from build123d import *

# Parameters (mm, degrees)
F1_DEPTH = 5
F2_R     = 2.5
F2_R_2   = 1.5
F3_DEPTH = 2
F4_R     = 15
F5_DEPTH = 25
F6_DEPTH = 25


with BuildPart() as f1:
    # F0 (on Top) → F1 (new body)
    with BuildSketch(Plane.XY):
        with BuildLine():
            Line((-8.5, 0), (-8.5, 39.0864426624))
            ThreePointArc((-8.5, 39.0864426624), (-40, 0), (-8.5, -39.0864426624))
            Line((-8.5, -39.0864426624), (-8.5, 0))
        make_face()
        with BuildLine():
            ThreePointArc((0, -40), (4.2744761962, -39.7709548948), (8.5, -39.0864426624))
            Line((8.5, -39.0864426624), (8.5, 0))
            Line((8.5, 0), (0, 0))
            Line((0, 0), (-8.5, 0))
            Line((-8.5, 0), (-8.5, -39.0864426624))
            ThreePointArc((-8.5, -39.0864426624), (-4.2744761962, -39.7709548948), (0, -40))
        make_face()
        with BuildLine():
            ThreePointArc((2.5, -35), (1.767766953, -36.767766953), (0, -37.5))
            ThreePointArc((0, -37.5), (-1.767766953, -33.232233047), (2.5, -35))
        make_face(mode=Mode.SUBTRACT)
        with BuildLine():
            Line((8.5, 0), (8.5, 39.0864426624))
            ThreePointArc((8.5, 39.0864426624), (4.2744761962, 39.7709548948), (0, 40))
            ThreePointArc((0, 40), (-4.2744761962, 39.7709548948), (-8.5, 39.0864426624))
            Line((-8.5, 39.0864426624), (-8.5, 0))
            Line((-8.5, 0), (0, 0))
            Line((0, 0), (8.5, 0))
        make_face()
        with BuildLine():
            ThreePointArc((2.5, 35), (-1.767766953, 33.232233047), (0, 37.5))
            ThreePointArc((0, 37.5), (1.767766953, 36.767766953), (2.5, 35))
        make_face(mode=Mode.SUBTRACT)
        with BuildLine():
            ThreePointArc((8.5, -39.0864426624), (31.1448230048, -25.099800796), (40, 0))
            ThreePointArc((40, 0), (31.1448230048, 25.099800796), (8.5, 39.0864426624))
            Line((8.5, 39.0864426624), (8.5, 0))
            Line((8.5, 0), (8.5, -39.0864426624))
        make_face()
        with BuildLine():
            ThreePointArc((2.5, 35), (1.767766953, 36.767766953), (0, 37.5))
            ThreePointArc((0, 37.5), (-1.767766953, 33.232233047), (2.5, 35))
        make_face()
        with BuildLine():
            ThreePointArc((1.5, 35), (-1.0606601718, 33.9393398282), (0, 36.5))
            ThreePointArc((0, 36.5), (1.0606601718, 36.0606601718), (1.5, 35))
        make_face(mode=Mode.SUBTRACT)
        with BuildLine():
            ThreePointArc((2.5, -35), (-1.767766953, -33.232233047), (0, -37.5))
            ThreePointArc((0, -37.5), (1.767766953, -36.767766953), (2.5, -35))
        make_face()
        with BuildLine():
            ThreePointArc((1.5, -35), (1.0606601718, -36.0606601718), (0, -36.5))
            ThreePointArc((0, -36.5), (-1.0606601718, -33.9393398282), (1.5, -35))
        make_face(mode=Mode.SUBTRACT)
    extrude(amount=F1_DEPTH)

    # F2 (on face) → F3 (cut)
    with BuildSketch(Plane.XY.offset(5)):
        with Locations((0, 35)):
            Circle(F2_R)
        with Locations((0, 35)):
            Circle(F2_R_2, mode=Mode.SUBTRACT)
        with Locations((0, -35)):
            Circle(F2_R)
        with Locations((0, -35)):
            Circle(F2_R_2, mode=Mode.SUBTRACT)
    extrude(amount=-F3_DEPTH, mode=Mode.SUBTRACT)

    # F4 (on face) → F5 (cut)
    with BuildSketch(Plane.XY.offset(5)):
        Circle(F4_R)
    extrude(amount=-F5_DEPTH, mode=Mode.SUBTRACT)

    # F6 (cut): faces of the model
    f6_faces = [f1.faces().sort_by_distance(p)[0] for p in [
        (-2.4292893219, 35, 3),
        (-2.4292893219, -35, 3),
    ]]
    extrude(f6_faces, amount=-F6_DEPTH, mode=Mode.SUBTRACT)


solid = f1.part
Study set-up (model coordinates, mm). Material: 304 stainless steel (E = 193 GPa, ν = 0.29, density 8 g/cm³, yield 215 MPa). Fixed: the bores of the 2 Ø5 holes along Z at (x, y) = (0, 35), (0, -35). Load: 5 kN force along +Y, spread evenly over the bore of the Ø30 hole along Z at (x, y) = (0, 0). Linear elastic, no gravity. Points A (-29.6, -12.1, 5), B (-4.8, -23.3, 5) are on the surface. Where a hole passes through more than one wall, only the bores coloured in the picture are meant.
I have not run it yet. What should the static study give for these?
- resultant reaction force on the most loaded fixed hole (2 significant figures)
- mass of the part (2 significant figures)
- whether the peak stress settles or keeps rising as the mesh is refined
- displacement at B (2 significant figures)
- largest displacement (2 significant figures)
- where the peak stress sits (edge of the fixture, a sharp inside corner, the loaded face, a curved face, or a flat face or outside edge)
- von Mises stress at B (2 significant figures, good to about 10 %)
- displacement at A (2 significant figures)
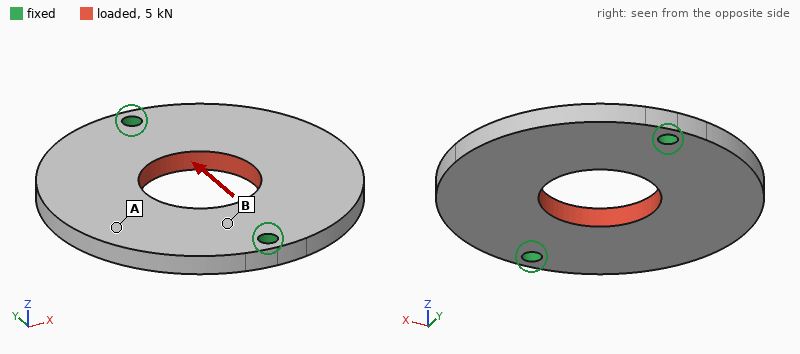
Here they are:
2.5 kN
170 g
keeps rising
1.8 µm
4.1 µm
edge of the fixture
23 MPa
3.1 µm
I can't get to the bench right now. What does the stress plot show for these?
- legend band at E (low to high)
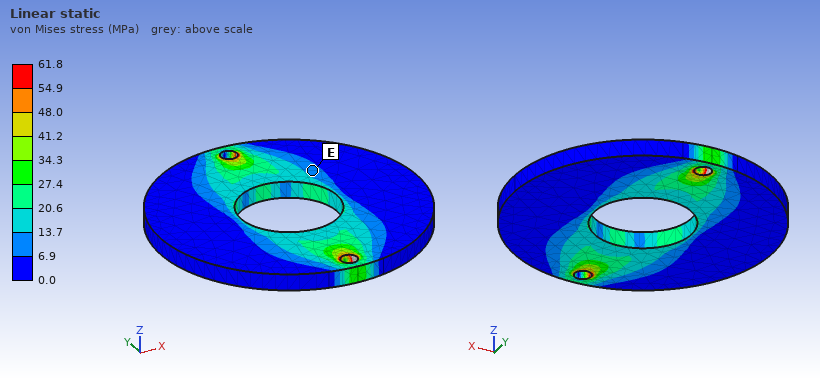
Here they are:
6.9 to 13.7 MPa
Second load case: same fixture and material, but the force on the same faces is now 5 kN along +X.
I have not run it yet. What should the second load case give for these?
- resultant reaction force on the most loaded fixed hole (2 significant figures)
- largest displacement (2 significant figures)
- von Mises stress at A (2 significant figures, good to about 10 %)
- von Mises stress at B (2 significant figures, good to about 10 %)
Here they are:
2.5 kN
4.9 µm
11 MPa
16 MPa
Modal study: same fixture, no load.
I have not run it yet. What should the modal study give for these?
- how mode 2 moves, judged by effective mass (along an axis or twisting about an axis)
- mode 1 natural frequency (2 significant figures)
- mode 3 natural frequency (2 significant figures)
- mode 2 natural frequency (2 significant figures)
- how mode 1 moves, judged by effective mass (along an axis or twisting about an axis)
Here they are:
along Z
1900 Hz
5600 Hz
2400 Hz
twisting about Y
